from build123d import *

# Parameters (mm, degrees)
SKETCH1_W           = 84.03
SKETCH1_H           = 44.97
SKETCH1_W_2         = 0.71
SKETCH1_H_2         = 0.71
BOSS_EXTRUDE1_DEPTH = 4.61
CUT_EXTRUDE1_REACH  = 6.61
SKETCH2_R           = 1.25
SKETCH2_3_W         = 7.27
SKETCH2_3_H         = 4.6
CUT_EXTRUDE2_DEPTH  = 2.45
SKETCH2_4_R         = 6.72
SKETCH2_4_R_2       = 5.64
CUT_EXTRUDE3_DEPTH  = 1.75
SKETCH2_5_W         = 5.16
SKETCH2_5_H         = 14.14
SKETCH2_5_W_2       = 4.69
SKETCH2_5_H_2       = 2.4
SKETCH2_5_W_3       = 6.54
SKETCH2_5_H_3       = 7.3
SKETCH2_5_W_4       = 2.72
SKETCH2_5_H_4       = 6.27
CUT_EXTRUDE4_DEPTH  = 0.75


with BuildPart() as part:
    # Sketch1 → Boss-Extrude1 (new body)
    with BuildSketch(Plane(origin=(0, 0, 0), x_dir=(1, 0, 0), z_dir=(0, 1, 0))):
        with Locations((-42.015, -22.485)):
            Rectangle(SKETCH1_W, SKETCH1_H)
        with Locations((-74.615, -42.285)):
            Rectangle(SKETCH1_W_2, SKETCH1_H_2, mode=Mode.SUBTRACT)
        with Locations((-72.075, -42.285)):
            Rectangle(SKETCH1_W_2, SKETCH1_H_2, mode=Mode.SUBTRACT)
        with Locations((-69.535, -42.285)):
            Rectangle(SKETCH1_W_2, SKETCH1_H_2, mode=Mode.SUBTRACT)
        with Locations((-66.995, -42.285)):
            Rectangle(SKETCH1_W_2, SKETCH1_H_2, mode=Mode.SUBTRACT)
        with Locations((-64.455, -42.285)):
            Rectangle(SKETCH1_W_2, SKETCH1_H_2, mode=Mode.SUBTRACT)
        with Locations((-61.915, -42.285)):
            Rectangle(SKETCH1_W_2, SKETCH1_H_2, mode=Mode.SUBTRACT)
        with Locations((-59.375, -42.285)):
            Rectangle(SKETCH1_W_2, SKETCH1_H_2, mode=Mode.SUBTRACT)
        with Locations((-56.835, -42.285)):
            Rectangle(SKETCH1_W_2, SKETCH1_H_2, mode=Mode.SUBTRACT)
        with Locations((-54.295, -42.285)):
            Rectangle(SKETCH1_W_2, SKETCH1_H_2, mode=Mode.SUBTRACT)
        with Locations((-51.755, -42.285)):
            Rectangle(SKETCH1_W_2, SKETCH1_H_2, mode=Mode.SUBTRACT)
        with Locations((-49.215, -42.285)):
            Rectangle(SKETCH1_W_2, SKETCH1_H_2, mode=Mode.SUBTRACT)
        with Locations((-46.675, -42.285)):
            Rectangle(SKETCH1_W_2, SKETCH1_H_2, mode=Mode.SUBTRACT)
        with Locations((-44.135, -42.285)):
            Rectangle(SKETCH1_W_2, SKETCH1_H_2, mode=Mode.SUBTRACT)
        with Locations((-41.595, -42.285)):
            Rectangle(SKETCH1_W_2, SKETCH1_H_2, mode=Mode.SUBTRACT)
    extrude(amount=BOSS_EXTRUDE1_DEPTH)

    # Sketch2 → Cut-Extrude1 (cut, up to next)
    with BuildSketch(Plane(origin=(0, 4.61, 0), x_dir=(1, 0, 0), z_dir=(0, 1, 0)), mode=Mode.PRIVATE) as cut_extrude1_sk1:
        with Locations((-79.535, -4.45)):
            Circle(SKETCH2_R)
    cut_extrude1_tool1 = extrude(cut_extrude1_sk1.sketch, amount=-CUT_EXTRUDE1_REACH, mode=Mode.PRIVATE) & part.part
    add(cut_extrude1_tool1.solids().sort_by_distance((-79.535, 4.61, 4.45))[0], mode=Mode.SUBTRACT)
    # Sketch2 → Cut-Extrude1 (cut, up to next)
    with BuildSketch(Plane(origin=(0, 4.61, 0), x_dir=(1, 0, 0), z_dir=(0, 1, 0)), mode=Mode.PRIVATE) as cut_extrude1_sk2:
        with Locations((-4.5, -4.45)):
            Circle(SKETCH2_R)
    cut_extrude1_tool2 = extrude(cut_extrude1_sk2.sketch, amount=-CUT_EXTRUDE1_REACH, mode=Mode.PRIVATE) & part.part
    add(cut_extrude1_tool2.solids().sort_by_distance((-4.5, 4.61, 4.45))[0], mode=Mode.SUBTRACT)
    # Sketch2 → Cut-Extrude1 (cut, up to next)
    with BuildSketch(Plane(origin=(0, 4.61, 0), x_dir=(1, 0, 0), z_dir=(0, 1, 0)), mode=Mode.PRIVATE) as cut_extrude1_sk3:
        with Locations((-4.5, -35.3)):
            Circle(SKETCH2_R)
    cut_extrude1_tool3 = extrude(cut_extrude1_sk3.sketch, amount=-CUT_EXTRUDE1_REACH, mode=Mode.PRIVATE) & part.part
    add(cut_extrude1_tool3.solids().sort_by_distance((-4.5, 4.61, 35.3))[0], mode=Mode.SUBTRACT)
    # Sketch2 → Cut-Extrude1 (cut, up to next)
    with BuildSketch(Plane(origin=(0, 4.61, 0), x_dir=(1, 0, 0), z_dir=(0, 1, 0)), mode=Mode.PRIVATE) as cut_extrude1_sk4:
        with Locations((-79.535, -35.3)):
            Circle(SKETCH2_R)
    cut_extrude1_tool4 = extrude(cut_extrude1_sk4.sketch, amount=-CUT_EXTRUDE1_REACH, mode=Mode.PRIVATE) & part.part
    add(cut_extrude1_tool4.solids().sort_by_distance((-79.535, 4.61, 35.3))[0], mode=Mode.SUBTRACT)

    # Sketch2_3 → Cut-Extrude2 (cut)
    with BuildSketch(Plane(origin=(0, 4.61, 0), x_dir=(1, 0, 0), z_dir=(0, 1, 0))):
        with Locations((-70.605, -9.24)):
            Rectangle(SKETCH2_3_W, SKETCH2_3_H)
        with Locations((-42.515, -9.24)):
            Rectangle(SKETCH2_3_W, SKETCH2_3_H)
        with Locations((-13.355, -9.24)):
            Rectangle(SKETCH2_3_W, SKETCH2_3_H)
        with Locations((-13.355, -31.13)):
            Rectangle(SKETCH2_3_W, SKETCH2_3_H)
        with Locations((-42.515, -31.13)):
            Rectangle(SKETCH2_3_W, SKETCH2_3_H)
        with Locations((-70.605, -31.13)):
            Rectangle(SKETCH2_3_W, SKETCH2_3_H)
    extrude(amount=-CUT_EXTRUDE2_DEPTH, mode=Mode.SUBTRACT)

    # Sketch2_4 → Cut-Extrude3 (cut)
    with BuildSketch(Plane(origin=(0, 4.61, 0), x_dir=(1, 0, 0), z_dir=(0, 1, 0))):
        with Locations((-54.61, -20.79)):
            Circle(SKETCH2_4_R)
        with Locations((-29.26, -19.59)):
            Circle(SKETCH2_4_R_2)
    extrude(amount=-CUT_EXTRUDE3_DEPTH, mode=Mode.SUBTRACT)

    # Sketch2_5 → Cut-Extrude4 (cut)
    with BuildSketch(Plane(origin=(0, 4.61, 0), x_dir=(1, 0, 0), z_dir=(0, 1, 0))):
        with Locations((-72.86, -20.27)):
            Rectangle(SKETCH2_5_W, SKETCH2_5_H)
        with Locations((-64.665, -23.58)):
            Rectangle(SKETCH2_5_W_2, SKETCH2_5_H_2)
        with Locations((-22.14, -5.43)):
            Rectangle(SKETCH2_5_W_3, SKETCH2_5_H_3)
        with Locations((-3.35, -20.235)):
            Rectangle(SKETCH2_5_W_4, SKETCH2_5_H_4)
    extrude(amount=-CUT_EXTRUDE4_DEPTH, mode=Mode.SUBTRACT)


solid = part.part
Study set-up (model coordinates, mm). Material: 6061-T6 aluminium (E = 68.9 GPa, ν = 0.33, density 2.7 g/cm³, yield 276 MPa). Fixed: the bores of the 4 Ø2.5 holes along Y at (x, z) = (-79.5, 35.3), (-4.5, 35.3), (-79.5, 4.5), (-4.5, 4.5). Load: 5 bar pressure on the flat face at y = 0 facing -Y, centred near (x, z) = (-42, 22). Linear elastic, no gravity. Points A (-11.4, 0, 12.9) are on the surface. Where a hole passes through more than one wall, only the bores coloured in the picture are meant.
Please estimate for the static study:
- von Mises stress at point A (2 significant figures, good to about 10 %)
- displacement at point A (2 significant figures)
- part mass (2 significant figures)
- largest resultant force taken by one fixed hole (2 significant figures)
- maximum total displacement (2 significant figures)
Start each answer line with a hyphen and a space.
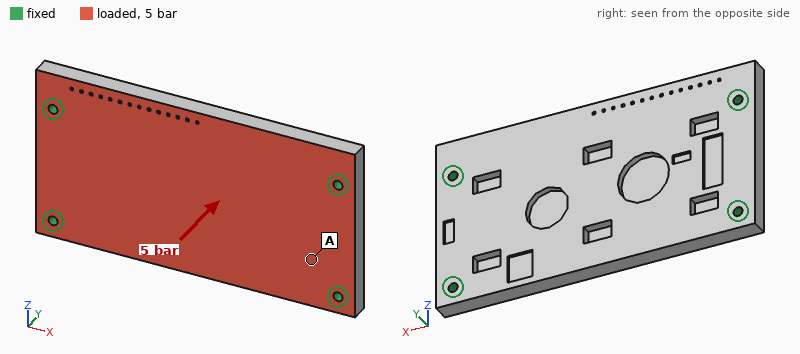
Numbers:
- 23 MPa
- 0.024 mm
- 44 g
- 540 N
- 0.12 mm
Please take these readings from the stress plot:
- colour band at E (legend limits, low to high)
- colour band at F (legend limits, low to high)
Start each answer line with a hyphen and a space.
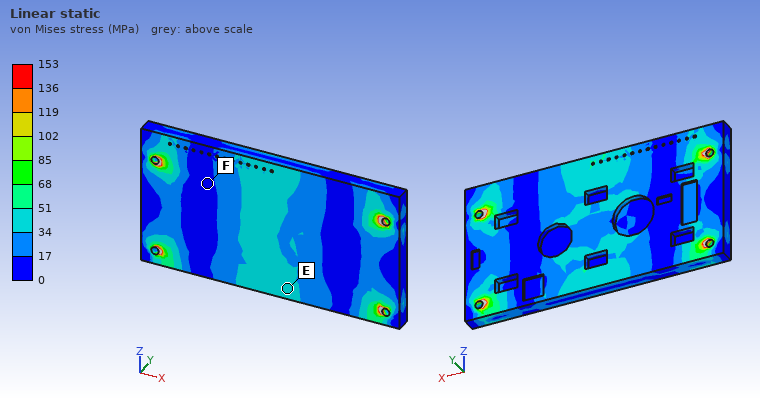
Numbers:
- 34 to 51 MPa
- 0 to 17 MPa
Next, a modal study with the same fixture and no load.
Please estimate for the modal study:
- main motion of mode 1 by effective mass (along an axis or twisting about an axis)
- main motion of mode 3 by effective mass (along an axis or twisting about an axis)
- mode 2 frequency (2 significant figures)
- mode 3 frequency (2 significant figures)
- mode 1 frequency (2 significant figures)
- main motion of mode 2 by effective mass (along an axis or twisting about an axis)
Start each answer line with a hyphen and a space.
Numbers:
- along Y
- twisting about Z
- 5500 Hz
- 9600 Hz
- 3600 Hz
- twisting about X
